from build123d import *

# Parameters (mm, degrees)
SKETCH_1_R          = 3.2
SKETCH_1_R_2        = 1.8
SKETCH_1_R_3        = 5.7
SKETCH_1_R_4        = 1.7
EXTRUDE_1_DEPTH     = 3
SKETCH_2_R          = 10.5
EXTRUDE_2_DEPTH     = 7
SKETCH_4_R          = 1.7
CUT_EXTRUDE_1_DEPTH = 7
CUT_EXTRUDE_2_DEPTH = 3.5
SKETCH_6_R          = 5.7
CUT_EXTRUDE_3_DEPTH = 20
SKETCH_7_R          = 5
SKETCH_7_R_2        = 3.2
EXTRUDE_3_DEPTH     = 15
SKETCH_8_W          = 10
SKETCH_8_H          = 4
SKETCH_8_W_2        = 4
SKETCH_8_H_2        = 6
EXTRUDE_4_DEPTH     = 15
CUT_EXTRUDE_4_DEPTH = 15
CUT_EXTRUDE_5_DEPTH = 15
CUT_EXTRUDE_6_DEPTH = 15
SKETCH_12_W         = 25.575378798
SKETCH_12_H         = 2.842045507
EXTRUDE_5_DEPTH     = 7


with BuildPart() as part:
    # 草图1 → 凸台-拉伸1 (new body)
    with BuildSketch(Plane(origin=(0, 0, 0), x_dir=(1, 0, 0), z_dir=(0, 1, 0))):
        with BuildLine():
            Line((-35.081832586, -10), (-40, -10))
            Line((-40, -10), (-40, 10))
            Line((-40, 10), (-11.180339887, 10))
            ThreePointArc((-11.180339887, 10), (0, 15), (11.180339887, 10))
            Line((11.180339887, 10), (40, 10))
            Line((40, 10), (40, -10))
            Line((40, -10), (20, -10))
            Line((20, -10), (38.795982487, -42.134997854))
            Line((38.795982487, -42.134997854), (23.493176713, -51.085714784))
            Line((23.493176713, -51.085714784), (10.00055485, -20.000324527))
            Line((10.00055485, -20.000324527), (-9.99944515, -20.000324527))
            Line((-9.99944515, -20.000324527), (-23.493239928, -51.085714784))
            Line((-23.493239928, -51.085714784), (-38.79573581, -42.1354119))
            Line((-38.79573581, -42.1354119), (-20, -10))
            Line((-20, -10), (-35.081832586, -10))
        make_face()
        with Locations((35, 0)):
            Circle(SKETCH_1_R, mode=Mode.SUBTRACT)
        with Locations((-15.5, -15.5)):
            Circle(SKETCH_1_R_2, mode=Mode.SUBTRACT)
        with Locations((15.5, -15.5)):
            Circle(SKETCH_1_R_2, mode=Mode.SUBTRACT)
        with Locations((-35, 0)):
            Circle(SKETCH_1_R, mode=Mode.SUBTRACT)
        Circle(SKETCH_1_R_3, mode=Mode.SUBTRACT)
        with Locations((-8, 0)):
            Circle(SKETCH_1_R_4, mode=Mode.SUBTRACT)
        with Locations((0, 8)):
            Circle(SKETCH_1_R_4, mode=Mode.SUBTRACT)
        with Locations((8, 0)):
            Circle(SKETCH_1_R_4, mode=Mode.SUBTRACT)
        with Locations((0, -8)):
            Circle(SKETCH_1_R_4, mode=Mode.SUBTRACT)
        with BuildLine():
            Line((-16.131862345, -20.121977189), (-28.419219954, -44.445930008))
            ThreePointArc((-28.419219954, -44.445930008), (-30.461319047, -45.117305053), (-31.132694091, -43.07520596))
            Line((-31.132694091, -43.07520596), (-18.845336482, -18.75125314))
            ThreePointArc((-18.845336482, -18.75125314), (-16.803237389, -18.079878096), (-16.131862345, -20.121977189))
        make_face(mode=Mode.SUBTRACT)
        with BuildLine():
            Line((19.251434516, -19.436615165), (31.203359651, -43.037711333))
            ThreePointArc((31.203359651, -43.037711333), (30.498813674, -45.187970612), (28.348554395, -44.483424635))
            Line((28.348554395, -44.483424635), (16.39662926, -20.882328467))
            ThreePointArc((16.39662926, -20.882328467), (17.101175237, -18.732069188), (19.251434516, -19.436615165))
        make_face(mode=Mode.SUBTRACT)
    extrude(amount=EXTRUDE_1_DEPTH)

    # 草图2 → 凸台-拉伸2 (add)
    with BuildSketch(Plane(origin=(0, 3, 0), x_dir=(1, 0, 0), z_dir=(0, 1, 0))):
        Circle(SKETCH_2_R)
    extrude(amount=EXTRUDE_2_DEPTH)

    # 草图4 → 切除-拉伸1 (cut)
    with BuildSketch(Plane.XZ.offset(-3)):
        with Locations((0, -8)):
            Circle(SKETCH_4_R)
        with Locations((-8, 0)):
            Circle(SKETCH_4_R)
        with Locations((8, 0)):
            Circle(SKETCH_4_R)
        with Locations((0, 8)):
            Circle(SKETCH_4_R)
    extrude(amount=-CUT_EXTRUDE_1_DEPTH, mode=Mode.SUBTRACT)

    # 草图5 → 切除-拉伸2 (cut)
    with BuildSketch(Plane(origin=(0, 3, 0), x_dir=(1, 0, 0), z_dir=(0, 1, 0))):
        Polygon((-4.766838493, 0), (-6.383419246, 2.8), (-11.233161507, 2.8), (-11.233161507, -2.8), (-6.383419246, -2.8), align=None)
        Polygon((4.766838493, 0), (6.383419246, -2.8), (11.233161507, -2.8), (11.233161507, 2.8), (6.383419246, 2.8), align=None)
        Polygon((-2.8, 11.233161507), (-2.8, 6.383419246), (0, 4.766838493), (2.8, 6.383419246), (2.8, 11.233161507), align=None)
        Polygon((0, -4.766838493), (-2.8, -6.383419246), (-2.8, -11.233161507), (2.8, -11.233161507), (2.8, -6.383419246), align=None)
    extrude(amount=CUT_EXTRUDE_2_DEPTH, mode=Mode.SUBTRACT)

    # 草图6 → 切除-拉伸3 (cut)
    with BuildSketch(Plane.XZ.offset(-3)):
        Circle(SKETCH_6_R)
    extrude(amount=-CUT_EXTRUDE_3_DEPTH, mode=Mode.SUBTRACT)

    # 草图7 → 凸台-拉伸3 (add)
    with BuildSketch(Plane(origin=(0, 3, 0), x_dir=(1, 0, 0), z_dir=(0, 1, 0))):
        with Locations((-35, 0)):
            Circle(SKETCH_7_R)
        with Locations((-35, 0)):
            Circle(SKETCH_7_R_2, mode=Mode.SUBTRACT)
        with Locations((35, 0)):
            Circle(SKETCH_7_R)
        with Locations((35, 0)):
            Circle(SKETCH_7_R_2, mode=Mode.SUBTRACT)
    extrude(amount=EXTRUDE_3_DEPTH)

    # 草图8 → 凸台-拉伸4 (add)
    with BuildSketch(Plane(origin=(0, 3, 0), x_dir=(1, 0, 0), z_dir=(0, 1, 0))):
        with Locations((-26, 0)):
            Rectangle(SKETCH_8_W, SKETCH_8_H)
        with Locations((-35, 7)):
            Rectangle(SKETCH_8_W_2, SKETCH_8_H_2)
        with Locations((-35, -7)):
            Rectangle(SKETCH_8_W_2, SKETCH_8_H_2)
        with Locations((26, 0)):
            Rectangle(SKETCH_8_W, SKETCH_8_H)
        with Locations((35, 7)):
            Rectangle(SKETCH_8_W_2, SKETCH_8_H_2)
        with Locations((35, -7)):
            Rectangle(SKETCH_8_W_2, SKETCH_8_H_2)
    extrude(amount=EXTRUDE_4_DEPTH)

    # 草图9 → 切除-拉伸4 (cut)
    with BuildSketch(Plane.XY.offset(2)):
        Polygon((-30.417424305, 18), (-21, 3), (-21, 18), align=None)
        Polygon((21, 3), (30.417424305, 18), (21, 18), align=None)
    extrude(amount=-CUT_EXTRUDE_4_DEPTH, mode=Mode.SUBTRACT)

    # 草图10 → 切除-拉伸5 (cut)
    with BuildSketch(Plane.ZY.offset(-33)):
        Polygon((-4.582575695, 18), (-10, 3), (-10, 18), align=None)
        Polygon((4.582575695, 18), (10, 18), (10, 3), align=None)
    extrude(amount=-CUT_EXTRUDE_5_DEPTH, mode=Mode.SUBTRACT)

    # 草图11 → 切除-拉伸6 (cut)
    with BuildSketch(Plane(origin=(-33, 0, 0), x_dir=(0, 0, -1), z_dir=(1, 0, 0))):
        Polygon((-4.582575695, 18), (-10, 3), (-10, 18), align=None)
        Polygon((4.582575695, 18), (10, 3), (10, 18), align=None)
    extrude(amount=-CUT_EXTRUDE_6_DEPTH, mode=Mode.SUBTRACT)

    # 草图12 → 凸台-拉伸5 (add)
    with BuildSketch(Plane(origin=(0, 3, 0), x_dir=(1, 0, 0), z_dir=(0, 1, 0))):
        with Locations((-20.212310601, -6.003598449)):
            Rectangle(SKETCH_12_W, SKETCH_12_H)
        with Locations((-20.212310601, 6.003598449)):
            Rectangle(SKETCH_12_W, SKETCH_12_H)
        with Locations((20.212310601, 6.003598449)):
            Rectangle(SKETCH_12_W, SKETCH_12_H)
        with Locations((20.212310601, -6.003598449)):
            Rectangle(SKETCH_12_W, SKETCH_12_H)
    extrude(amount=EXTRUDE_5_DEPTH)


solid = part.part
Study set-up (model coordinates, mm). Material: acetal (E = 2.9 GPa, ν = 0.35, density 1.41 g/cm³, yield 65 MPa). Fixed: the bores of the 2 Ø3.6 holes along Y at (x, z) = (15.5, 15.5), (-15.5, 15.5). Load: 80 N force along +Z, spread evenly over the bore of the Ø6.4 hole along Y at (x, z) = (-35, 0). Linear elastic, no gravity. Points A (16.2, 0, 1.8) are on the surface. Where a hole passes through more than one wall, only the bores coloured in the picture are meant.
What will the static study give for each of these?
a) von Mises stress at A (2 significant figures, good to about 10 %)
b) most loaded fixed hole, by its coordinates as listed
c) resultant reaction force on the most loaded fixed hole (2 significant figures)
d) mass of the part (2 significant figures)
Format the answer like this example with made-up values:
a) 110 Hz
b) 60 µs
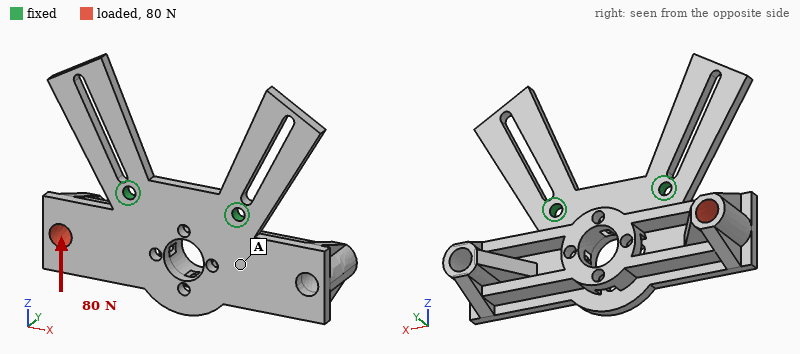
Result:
a) 3.2 MPa
b) (-15.5, 15.5)
c) 130 N
d) 19 g
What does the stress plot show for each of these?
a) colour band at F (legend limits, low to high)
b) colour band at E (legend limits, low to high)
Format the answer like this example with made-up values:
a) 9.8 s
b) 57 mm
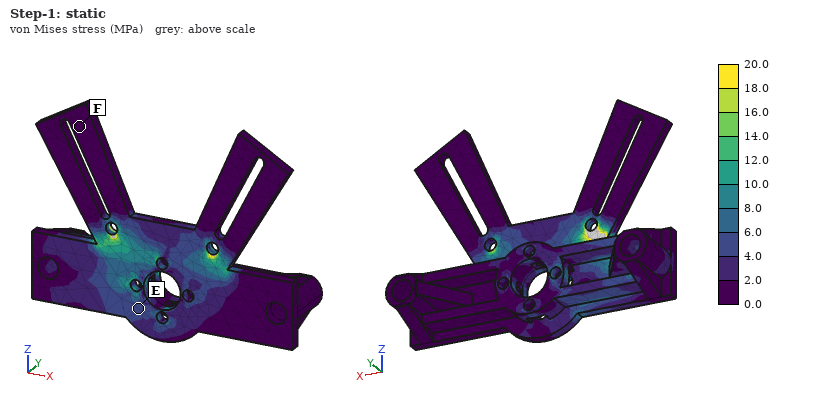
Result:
a) 0.0 to 2.0 MPa
b) 4.0 to 6.0 MPa
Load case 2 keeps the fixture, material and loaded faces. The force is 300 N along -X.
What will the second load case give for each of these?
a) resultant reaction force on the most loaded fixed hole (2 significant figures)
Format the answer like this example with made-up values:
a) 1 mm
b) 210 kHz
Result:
a) 210 N
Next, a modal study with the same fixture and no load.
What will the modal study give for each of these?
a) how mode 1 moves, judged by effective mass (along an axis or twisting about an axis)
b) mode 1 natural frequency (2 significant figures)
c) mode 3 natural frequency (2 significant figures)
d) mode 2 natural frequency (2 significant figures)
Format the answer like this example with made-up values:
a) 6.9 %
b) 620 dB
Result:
a) along Y
b) 480 Hz
c) 530 Hz
d) 520 Hz
